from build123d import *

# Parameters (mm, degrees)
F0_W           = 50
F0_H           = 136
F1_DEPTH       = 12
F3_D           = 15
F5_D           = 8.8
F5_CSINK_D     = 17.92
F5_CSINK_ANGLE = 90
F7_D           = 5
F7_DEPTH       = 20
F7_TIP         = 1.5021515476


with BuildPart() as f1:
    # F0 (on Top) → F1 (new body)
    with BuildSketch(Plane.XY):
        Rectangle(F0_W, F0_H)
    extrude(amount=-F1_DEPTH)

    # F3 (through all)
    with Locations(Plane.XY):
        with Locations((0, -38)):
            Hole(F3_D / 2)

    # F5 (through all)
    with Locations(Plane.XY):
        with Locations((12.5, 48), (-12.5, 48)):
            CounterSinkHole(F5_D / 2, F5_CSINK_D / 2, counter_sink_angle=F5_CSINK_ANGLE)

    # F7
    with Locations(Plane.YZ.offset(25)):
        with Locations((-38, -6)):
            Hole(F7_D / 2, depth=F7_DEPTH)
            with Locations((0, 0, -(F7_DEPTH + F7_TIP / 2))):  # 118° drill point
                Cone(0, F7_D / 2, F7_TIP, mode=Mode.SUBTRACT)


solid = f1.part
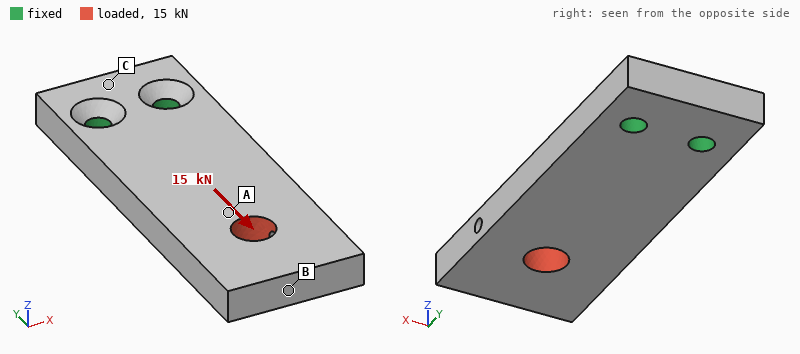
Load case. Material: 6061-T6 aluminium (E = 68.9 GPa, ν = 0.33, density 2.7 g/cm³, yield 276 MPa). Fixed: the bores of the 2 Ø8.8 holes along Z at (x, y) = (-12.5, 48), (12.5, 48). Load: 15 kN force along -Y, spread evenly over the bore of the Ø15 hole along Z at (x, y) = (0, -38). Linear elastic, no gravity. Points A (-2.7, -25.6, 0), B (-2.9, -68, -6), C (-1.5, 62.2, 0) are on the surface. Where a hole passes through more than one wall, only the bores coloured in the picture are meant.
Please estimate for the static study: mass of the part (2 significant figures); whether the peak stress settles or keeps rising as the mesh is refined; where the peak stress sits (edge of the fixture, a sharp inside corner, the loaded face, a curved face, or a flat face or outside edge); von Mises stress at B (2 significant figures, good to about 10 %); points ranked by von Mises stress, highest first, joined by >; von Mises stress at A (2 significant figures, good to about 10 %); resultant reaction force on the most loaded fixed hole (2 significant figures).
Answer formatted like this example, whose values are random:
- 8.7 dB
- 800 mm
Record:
- 210 g
- keeps rising
- edge of the fixture
- 18 MPa
- A > B > C
- 32 MPa
- 7.7 kN
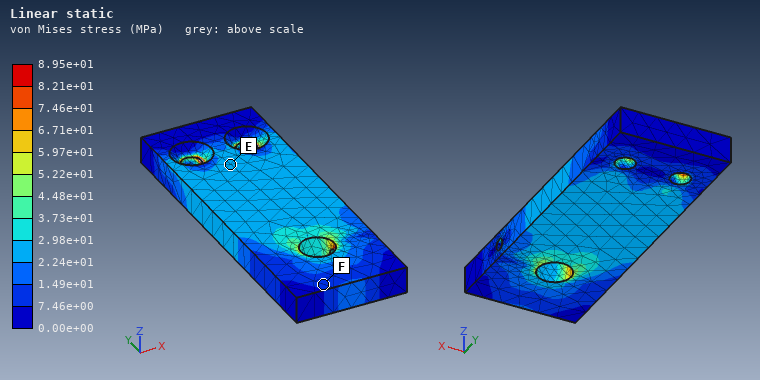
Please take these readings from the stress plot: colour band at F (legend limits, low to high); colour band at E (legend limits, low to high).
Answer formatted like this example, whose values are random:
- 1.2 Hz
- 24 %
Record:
- 7.46e+00 to 1.49e+01 MPa
- 2.24e+01 to 2.98e+01 MPa
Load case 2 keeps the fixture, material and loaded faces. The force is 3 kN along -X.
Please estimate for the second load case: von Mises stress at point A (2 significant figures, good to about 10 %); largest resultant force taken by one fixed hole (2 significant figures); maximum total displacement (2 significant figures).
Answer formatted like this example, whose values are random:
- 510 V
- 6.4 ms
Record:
- 17 MPa
- 8.6 kN
- 0.17 mm
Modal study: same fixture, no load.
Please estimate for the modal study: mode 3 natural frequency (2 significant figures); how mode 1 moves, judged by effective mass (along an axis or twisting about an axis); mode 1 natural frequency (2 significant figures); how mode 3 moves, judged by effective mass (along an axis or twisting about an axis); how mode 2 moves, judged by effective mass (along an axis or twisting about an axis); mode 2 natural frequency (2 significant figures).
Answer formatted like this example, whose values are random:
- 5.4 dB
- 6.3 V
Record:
- 3100 Hz
- along Z
- 690 Hz
- twisting about Y
- along X
- 2500 Hz
